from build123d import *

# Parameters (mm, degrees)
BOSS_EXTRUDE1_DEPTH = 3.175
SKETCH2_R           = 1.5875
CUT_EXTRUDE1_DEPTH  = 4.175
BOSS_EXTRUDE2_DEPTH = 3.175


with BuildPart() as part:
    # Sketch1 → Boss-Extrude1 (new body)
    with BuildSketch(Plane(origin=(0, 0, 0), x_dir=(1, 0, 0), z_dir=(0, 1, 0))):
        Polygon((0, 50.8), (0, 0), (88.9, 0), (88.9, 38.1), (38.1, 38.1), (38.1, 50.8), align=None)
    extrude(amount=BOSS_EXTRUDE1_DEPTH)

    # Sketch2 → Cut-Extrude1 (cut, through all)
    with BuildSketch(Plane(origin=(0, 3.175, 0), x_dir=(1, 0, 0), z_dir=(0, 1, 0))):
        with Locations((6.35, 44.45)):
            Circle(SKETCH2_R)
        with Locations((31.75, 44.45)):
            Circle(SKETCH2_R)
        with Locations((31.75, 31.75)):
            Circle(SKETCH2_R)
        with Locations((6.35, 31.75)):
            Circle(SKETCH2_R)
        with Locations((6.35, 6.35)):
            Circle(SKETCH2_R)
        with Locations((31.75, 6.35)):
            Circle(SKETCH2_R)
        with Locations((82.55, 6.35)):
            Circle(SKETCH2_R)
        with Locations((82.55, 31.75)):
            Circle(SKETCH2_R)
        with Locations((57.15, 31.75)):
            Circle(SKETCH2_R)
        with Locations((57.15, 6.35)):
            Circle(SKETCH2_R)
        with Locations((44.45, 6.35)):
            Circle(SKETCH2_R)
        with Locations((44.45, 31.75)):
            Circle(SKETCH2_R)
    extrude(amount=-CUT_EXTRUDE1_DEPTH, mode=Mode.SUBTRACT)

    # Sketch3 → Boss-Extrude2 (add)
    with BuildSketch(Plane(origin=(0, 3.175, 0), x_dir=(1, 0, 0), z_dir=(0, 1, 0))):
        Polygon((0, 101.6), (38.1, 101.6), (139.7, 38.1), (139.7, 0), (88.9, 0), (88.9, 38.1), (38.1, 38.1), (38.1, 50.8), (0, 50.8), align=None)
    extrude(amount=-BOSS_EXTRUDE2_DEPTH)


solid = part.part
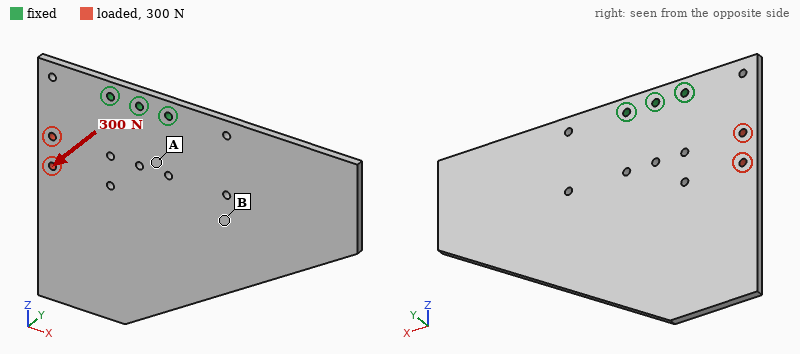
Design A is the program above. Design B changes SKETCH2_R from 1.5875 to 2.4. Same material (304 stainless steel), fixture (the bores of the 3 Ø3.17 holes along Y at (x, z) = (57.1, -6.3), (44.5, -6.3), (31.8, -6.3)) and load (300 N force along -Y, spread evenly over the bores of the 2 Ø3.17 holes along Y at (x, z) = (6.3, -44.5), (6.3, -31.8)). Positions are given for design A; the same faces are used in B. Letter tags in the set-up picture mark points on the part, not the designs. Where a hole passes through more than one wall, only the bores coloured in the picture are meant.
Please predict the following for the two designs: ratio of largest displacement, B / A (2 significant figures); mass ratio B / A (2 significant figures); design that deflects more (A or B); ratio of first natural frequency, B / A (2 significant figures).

0.92
0.99
A
1.0
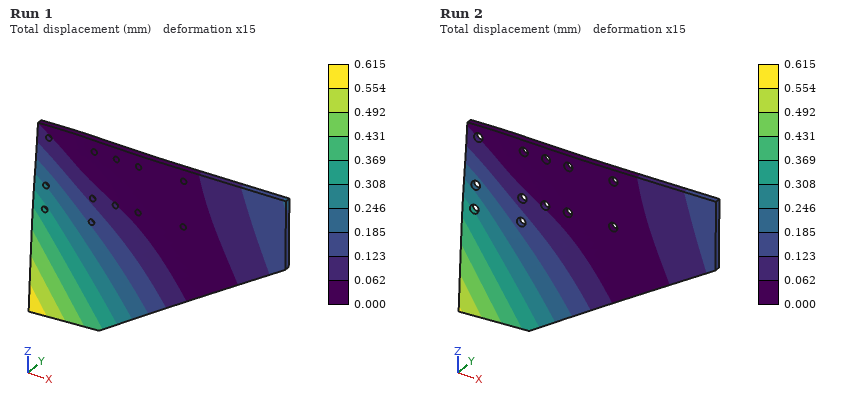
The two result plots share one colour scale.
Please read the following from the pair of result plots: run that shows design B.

Run 2
